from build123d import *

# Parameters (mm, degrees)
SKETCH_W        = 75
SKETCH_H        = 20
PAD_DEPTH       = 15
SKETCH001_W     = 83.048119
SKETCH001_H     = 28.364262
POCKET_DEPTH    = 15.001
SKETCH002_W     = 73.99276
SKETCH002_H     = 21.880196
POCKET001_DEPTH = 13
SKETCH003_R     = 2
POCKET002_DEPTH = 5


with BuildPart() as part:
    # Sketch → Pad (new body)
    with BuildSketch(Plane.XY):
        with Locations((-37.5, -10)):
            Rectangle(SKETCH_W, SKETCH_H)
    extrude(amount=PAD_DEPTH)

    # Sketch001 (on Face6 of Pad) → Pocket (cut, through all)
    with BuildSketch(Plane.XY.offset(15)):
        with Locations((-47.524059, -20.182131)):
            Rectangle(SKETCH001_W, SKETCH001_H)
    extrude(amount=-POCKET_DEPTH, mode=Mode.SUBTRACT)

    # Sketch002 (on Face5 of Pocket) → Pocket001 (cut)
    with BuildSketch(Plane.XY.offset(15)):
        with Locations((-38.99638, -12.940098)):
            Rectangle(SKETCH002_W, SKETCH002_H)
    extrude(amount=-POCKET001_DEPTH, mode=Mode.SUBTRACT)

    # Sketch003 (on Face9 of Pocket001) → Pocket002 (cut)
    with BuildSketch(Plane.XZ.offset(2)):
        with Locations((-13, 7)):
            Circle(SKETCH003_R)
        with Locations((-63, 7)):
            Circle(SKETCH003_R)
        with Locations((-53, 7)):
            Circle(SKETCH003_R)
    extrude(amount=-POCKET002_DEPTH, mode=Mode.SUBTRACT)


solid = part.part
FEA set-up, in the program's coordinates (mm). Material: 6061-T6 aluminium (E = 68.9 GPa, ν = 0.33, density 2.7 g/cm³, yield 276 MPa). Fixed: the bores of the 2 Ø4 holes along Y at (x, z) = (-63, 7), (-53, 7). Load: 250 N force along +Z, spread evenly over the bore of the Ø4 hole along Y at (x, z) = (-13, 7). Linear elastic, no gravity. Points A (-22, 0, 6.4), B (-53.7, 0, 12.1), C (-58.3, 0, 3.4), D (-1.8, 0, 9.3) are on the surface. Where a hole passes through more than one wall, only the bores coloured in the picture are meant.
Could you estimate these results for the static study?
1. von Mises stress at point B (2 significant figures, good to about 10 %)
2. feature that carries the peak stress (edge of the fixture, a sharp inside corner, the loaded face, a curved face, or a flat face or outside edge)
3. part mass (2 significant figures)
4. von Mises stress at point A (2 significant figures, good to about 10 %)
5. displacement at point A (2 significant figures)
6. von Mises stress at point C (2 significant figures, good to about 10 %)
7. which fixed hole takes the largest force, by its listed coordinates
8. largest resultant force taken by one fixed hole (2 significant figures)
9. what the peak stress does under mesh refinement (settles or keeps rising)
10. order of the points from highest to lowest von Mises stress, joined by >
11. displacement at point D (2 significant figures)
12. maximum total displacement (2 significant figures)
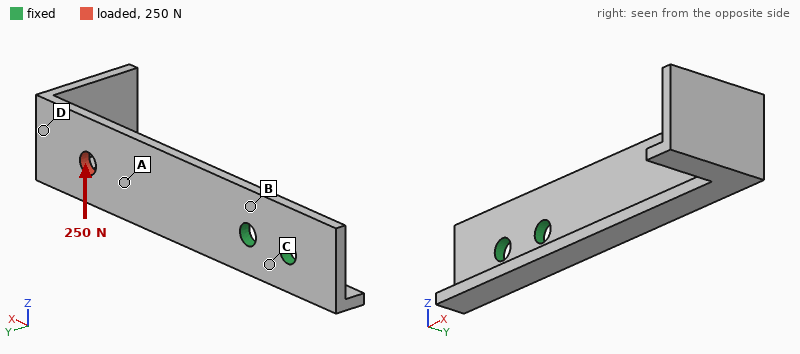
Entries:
61 MPa
edge of the fixture
9.2 g
21 MPa
0.18 mm
43 MPa
(-53, 7)
790 N
keeps rising
B > C > A > D
0.37 mm
0.44 mm
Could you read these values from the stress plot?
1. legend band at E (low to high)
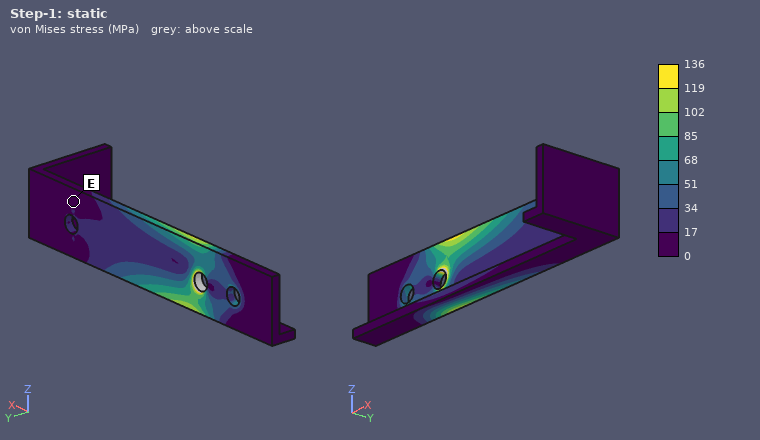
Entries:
0 to 17 MPa
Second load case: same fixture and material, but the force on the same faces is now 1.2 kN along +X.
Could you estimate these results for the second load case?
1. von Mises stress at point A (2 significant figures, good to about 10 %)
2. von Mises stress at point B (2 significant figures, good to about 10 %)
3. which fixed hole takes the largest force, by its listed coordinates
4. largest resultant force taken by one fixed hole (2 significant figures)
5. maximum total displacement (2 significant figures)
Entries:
51 MPa
23 MPa
(-53, 7)
970 N
0.20 mm
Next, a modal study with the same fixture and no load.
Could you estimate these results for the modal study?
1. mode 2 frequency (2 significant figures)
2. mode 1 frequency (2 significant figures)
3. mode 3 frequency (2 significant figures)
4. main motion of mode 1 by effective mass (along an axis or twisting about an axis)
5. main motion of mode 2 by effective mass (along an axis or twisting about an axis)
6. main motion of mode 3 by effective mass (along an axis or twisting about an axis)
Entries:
1300 Hz
740 Hz
3400 Hz
along Y
along Z
along Z
